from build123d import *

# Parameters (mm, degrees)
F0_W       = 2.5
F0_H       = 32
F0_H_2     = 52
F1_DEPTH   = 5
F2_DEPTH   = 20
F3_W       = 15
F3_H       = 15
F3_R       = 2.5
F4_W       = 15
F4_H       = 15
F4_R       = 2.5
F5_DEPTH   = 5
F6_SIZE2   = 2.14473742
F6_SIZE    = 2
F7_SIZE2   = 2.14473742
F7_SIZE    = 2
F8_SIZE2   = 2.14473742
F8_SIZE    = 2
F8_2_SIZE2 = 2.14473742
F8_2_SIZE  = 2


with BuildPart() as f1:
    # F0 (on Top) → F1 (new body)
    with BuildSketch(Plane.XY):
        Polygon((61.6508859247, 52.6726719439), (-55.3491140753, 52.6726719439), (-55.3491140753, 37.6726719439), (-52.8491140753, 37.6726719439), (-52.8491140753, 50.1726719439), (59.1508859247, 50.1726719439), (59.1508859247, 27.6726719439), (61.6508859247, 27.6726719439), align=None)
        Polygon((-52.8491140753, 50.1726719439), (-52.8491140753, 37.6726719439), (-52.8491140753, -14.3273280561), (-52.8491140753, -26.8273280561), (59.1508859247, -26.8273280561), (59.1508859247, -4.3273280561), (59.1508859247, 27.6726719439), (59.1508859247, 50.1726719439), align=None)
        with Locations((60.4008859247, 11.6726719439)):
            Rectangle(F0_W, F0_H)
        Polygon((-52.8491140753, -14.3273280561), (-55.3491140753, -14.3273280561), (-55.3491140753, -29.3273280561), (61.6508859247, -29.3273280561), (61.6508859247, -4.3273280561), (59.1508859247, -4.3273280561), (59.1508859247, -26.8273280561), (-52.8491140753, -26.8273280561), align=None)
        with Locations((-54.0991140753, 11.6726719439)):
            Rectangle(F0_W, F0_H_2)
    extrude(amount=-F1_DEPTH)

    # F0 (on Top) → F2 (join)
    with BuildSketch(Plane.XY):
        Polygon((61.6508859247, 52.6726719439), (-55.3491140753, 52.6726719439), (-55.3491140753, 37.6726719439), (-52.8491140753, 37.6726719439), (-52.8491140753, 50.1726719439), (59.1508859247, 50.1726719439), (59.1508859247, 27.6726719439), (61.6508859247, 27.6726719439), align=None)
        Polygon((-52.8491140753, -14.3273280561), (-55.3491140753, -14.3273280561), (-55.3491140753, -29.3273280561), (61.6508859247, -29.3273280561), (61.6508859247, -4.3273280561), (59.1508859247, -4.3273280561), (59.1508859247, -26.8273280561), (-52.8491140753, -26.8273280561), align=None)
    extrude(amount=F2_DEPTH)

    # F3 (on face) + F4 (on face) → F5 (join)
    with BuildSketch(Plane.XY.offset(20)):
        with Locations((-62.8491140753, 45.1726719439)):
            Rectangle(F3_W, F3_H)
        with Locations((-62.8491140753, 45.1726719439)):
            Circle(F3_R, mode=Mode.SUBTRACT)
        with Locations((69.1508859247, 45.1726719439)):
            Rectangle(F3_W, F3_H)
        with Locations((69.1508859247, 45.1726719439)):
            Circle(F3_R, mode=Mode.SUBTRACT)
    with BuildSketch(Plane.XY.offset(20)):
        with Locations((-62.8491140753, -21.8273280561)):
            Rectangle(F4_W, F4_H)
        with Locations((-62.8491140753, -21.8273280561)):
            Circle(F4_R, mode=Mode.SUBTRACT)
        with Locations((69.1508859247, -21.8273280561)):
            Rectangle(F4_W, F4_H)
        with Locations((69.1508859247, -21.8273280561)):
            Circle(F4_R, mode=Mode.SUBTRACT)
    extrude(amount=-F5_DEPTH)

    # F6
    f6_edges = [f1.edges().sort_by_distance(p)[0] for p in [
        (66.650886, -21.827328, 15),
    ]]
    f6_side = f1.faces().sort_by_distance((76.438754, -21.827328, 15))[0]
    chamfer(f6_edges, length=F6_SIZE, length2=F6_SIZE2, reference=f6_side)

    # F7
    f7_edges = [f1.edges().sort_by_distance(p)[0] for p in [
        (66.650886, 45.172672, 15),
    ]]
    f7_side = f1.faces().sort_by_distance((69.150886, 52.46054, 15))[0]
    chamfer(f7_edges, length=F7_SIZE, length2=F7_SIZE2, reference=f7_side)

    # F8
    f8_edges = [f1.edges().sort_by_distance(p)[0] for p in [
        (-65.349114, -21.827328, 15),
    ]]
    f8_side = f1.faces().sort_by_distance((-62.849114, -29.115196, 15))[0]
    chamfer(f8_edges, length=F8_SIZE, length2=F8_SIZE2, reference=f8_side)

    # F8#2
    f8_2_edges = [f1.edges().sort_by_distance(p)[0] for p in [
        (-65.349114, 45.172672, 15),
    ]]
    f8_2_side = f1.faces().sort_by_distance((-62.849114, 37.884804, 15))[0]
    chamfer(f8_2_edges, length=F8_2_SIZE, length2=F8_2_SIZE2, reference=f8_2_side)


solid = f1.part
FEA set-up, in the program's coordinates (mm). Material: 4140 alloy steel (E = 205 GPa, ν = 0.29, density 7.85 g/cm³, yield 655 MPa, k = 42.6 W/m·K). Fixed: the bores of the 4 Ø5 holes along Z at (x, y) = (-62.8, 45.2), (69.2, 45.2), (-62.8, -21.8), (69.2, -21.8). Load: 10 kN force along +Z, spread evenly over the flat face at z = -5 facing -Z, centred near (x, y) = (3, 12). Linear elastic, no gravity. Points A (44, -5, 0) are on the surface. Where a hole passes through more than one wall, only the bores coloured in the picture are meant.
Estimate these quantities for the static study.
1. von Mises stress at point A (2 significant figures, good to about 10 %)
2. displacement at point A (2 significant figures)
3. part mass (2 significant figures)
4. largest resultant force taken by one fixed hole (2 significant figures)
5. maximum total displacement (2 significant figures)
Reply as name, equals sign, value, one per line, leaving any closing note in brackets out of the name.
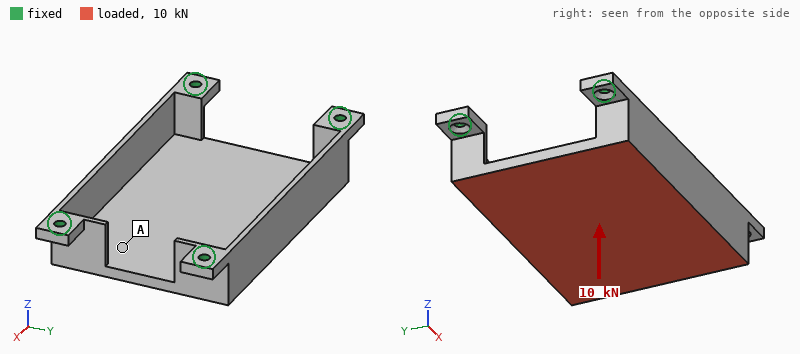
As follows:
von Mises stress at point A = 54 MPa
displacement at point A = 0.080 mm
part mass = 530 g
largest resultant force taken by one fixed hole = 3.3 kN
maximum total displacement = 0.18 mm
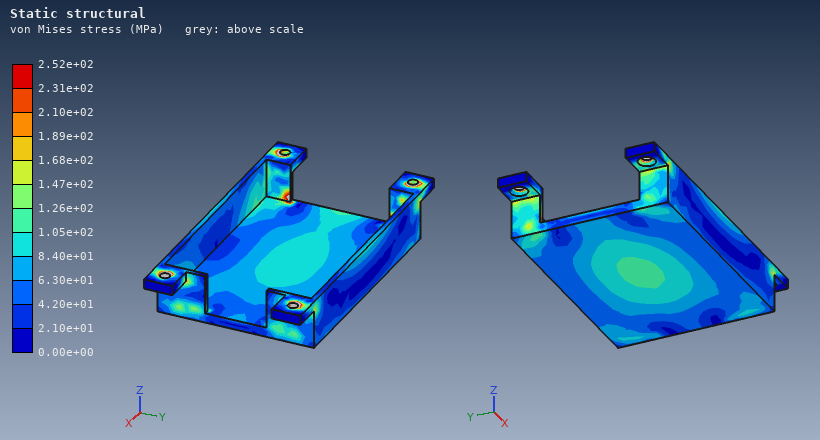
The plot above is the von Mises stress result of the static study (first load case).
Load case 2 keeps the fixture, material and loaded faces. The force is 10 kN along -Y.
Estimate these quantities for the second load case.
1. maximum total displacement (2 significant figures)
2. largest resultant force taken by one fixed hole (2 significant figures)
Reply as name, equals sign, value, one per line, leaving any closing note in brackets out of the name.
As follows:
maximum total displacement = 0.14 mm
largest resultant force taken by one fixed hole = 3.4 kN
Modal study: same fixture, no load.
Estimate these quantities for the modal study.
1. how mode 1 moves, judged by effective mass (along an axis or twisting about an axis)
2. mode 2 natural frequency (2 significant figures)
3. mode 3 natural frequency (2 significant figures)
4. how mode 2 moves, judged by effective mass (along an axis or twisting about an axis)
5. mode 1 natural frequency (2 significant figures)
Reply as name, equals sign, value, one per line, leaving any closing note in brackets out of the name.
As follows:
how mode 1 moves, judged by effective mass = along Y
mode 2 natural frequency = 2300 Hz
mode 3 natural frequency = 4200 Hz
how mode 2 moves, judged by effective mass = along Z
mode 1 natural frequency = 2200 Hz
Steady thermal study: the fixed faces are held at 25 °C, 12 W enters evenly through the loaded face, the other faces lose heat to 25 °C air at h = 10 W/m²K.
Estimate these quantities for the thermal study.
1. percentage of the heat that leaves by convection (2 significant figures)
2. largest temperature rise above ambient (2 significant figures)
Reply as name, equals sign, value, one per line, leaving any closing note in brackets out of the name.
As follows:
percentage of the heat that leaves by convection = 35 %
largest temperature rise above ambient = 23 K
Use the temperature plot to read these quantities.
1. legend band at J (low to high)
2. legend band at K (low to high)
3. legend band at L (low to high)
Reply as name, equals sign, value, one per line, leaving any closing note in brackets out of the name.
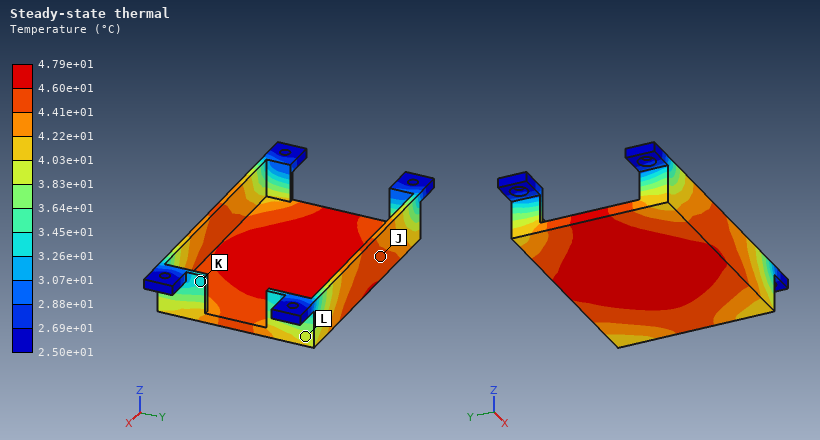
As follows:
legend band at J = 4.41e+01 to 4.60e+01 °C
legend band at K = 3.26e+01 to 3.45e+01 °C
legend band at L = 3.83e+01 to 4.03e+01 °C
